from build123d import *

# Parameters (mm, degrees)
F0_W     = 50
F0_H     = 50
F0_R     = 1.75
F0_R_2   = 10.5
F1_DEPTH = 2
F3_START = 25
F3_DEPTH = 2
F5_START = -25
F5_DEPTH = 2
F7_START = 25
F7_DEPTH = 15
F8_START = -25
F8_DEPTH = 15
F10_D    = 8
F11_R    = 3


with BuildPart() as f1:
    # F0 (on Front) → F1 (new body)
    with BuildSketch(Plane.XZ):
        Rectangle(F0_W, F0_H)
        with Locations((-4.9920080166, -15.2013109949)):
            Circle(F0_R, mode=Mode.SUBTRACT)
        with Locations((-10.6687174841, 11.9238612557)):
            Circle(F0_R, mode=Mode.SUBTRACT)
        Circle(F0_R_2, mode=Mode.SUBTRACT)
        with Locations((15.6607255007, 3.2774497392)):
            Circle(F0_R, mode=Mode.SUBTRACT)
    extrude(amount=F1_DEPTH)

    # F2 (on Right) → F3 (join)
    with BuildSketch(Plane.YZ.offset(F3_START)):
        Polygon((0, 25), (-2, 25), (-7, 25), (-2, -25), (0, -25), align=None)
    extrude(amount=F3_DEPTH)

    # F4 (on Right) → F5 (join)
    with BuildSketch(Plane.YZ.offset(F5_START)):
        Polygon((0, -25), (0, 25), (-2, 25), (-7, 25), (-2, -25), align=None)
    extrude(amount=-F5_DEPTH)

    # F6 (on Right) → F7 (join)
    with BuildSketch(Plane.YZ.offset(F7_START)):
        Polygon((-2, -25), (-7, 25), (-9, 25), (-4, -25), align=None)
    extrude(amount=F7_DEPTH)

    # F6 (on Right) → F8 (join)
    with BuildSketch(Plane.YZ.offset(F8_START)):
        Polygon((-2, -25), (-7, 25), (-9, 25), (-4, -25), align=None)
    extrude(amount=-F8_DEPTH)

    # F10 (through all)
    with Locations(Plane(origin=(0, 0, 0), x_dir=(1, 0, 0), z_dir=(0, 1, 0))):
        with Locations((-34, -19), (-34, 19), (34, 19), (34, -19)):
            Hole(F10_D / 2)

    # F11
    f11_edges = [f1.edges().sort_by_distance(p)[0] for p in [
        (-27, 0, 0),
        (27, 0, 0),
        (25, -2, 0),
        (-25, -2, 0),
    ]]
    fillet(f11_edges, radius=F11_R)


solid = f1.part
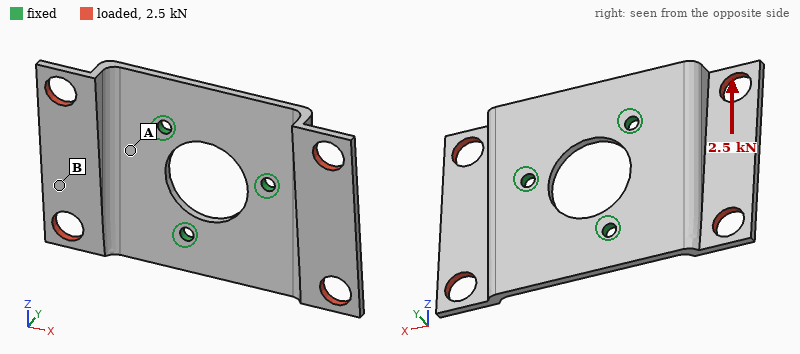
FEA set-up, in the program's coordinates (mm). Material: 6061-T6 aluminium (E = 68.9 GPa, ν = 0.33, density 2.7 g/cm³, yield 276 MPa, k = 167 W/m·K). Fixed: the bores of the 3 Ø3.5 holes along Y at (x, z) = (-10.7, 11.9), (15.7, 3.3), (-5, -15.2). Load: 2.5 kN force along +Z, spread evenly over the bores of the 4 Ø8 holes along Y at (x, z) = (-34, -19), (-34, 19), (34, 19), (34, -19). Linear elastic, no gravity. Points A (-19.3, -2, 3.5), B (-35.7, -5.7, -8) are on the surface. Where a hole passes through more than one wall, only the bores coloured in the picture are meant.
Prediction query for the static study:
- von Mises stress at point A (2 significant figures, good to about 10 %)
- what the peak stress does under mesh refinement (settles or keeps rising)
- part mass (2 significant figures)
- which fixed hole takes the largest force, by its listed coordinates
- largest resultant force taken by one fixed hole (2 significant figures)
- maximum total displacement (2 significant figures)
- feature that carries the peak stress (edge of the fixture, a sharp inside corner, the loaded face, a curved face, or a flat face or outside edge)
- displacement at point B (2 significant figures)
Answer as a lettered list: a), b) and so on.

a) 67 MPa
b) keeps rising
c) 21 g
d) (15.7, 3.3)
e) 1.2 kN
f) 0.32 mm
g) edge of the fixture
h) 0.15 mm
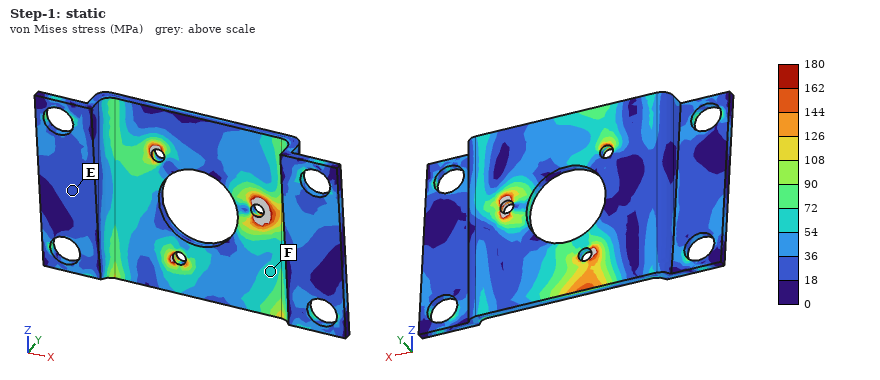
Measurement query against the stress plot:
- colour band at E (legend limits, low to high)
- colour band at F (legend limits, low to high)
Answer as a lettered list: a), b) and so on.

a) 18 to 36 MPa
b) 54 to 72 MPa
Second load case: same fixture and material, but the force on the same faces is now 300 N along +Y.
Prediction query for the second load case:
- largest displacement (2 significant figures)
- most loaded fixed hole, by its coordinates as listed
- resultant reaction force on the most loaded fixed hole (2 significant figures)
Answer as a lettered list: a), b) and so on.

a) 0.64 mm
b) (15.7, 3.3)
c) 210 N
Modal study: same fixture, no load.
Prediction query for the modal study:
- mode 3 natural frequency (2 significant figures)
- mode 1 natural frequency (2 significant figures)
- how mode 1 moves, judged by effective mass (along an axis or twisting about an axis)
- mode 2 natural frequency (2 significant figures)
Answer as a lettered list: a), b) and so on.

a) 2600 Hz
b) 1600 Hz
c) along Y
d) 2200 Hz
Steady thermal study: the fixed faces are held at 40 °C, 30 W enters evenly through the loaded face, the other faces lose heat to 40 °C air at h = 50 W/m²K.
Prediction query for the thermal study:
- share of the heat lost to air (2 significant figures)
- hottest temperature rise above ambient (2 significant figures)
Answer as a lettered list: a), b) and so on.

a) 19 %
b) 36 K
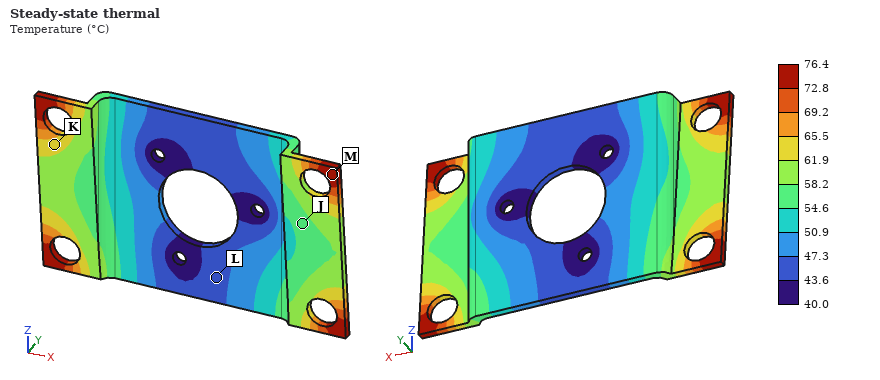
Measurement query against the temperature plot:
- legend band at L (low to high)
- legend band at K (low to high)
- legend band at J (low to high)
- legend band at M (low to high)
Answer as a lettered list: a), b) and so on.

a) 43.6 to 47.3 °C
b) 61.9 to 65.5 °C
c) 54.6 to 58.2 °C
d) 72.8 to 76.4 °C
